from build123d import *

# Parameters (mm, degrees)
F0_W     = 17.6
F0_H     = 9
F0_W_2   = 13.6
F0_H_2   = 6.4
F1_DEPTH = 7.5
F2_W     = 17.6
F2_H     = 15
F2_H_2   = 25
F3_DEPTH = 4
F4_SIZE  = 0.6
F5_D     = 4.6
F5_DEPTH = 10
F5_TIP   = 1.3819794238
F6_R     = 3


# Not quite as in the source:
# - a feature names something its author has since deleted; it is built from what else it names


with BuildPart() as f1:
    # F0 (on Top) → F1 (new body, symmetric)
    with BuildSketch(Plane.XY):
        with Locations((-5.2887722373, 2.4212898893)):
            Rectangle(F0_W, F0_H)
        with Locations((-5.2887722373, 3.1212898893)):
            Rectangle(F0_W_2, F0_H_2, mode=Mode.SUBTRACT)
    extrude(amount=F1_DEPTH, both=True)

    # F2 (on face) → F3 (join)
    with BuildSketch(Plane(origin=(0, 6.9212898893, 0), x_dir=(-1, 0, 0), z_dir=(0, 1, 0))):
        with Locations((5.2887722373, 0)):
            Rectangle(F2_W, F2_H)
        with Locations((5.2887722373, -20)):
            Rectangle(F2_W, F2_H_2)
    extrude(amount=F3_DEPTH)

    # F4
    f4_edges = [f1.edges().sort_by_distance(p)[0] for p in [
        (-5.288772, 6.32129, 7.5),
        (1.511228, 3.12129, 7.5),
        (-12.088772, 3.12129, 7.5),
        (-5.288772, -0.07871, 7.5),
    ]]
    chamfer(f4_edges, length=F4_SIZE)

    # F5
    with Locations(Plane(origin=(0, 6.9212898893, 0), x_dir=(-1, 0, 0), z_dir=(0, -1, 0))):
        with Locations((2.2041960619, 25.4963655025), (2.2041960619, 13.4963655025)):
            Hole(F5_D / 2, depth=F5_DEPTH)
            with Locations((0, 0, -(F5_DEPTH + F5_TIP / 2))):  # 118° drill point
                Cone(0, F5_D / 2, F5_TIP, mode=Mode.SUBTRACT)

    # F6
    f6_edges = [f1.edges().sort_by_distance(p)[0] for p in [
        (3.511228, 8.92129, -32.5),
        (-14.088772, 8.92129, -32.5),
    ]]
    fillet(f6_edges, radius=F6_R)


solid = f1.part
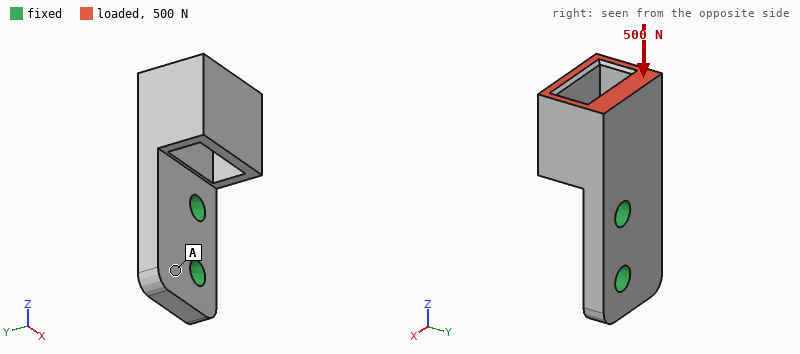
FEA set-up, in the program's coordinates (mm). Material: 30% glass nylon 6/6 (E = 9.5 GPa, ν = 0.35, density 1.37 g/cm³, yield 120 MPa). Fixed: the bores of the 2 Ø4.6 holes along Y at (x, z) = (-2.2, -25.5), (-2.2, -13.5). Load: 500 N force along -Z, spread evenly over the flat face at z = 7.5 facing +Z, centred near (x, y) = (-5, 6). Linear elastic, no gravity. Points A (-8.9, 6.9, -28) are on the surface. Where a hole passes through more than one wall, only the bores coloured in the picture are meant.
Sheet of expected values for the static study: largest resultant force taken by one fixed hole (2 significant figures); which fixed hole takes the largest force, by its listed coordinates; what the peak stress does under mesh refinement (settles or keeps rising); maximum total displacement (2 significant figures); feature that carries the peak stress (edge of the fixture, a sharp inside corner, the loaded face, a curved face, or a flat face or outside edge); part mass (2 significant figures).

410 N
(-2.2, -13.5)
keeps rising
0.32 mm
edge of the fixture
5.1 g
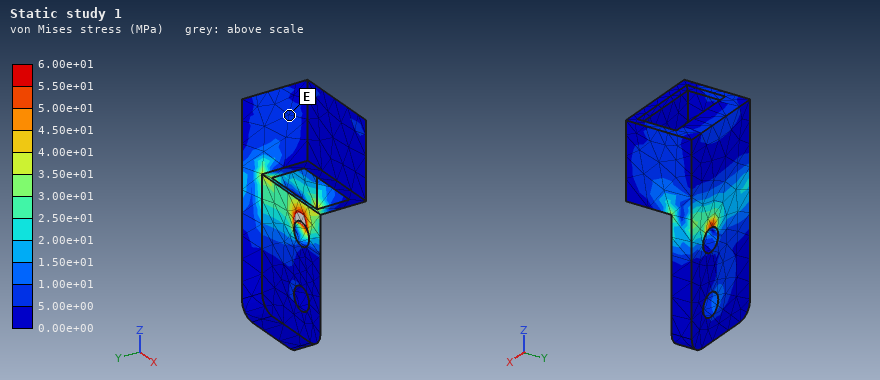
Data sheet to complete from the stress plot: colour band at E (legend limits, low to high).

5.00e+00 to 1.00e+01 MPa
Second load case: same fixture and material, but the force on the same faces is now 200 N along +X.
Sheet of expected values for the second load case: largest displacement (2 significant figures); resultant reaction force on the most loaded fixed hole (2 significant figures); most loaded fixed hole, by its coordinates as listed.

0.14 mm
400 N
(-2.2, -13.5)
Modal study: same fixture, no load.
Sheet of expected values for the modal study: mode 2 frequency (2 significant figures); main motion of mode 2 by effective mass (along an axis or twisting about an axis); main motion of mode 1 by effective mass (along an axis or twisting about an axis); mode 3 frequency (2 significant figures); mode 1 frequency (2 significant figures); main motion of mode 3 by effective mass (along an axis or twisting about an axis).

4200 Hz
along X
along Y
7000 Hz
2600 Hz
along X
